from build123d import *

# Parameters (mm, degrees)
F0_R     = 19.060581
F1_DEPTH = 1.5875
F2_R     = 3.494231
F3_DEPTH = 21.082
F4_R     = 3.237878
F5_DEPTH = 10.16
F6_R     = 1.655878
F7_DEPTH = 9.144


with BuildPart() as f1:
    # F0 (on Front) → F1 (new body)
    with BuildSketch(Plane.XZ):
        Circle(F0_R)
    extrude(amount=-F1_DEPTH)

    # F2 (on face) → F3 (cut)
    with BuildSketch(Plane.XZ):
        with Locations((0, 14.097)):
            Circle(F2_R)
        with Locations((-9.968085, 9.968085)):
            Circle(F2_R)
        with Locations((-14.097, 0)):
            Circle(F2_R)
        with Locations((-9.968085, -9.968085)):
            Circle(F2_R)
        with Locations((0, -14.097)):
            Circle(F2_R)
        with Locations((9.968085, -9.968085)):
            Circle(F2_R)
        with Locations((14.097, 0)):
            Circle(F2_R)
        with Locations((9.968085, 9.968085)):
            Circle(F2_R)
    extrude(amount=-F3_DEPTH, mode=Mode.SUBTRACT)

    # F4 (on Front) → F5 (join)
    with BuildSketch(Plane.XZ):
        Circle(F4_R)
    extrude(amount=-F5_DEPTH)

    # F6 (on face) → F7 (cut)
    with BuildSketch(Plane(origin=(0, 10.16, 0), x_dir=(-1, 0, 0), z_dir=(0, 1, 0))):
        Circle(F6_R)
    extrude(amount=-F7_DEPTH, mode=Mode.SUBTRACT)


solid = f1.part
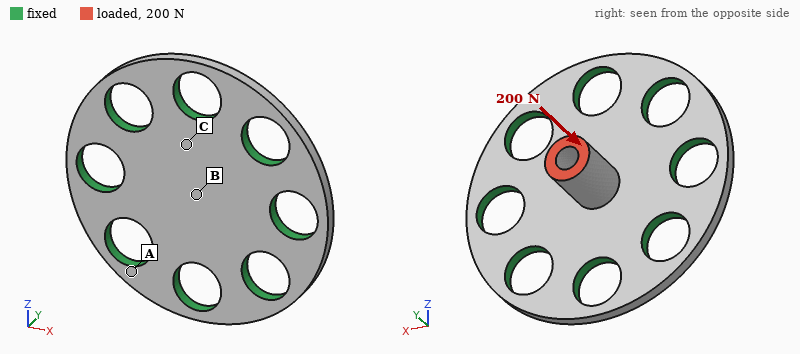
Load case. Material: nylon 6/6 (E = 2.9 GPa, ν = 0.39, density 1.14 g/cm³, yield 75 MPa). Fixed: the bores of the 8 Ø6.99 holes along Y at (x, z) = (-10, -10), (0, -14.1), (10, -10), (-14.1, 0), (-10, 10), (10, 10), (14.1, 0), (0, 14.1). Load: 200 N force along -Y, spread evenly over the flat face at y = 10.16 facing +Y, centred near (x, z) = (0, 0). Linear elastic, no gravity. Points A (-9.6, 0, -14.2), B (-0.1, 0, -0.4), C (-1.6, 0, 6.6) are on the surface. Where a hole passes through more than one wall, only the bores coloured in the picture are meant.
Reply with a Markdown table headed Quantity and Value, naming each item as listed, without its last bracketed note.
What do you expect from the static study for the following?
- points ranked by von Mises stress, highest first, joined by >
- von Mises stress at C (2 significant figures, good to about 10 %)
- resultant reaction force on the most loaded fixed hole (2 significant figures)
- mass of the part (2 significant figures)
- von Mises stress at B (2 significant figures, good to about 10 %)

| Quantity | Value |
|---|---|
| points ranked by von Mises stress, highest first, joined by > | B > C > A |
| von Mises stress at C | 14 MPa |
| resultant reaction force on the most loaded fixed hole | 27 N |
| mass of the part | 1.7 g |
| von Mises stress at B | 24 MPa |
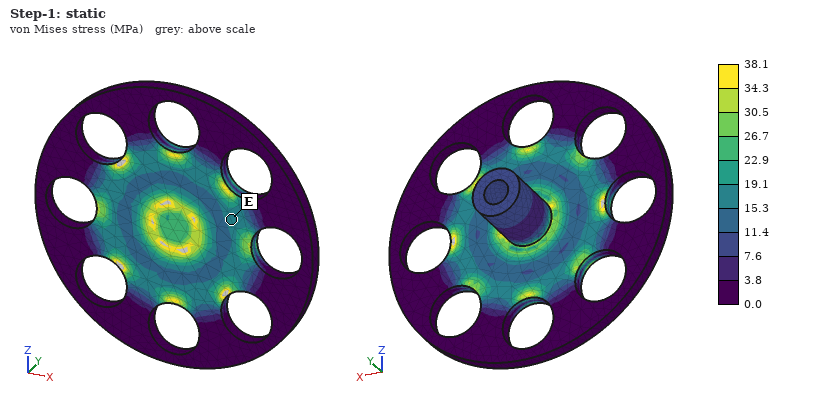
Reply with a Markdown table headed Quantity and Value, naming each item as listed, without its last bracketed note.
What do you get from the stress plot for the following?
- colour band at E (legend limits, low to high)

| Quantity | Value |
|---|---|
| colour band at E | 15.3 to 19.1 MPa |
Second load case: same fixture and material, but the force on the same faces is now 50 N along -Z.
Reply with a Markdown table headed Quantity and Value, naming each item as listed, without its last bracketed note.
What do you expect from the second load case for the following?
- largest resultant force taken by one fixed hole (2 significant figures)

| Quantity | Value |
|---|---|
| largest resultant force taken by one fixed hole | 20 N |
